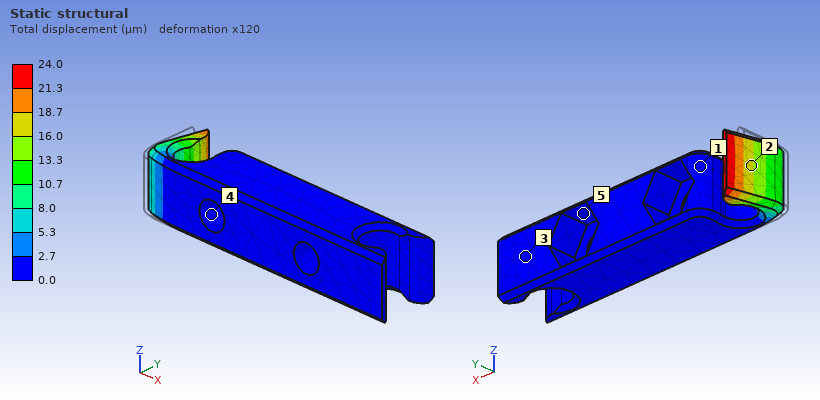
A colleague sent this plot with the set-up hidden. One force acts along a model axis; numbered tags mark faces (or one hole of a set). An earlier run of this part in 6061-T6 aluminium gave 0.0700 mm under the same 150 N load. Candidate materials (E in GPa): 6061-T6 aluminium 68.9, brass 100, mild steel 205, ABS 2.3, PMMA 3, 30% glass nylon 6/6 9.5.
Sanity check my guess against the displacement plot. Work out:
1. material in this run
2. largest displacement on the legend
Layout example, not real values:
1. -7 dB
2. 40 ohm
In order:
1. mild steel
2. 24.0 µm
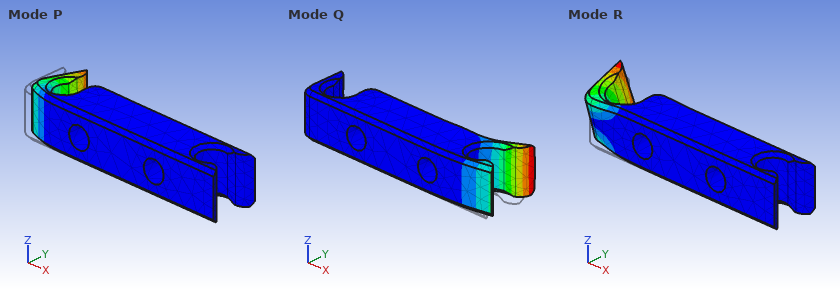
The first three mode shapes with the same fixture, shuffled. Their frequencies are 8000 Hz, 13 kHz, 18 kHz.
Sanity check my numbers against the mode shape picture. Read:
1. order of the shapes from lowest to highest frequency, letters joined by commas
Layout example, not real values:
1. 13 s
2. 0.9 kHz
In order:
1. P, R, Q
